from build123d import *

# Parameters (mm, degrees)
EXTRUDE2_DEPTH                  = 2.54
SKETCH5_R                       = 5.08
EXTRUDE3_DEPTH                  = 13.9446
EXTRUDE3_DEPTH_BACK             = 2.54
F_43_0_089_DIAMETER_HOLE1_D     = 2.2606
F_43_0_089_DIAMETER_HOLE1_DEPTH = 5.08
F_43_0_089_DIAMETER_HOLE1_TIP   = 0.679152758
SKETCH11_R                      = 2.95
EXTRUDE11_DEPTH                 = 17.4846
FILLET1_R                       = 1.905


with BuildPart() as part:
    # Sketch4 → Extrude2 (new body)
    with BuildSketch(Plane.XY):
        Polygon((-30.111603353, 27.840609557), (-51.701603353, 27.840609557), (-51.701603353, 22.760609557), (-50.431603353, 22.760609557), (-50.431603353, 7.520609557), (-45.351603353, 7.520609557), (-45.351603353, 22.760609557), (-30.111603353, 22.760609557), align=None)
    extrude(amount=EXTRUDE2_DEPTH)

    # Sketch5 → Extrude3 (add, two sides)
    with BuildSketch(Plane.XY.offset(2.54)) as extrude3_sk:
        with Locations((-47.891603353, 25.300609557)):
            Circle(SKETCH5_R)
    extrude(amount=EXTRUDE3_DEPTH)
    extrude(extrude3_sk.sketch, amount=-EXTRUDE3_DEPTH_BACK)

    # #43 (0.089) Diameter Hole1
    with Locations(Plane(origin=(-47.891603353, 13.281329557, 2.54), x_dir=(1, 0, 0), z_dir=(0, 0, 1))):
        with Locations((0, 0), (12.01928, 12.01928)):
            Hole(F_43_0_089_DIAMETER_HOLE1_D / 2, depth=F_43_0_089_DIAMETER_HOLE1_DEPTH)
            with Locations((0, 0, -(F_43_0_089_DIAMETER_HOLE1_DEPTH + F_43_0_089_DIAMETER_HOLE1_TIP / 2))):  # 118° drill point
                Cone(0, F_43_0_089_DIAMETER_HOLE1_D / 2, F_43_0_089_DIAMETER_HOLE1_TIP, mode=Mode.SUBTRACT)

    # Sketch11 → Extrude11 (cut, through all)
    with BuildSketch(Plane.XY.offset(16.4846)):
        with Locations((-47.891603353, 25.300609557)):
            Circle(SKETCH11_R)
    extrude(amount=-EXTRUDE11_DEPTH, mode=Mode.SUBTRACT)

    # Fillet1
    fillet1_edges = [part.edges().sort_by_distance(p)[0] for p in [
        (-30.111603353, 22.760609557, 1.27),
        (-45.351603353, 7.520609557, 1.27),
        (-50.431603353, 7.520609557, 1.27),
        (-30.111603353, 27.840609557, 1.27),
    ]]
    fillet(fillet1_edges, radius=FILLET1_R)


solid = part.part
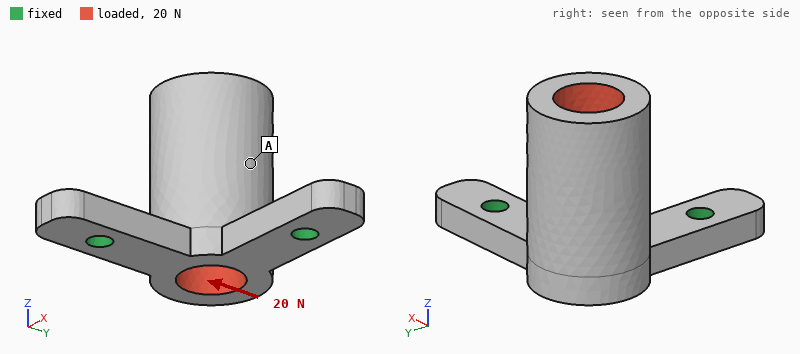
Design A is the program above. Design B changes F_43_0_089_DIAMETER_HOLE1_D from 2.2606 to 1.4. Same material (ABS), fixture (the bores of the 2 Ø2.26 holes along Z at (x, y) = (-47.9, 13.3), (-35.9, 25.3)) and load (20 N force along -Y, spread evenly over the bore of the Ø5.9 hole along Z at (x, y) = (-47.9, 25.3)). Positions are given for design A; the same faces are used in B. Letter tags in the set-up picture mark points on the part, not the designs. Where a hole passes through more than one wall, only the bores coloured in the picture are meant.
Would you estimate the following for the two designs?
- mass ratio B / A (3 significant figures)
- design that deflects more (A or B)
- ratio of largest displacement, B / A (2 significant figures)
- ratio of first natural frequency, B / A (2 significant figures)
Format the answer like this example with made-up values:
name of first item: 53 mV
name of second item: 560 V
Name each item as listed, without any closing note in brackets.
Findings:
mass ratio B / A: 1.01
design that deflects more: B
ratio of largest displacement, B / A: 1.1
ratio of first natural frequency, B / A: 0.95
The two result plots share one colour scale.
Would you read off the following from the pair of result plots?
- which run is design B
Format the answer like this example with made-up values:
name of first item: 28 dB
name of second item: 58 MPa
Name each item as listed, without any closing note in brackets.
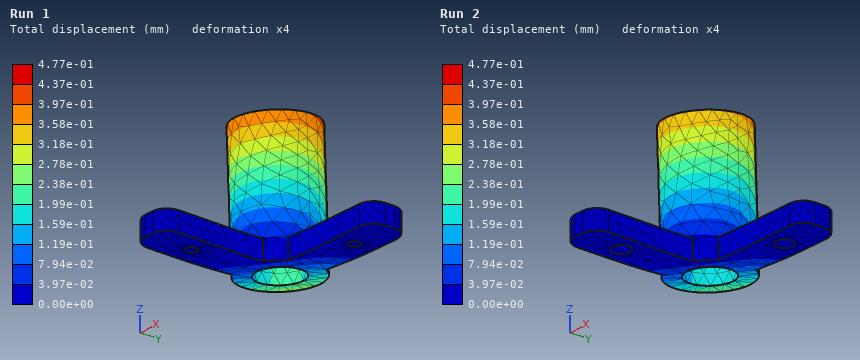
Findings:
which run is design B: Run 1
